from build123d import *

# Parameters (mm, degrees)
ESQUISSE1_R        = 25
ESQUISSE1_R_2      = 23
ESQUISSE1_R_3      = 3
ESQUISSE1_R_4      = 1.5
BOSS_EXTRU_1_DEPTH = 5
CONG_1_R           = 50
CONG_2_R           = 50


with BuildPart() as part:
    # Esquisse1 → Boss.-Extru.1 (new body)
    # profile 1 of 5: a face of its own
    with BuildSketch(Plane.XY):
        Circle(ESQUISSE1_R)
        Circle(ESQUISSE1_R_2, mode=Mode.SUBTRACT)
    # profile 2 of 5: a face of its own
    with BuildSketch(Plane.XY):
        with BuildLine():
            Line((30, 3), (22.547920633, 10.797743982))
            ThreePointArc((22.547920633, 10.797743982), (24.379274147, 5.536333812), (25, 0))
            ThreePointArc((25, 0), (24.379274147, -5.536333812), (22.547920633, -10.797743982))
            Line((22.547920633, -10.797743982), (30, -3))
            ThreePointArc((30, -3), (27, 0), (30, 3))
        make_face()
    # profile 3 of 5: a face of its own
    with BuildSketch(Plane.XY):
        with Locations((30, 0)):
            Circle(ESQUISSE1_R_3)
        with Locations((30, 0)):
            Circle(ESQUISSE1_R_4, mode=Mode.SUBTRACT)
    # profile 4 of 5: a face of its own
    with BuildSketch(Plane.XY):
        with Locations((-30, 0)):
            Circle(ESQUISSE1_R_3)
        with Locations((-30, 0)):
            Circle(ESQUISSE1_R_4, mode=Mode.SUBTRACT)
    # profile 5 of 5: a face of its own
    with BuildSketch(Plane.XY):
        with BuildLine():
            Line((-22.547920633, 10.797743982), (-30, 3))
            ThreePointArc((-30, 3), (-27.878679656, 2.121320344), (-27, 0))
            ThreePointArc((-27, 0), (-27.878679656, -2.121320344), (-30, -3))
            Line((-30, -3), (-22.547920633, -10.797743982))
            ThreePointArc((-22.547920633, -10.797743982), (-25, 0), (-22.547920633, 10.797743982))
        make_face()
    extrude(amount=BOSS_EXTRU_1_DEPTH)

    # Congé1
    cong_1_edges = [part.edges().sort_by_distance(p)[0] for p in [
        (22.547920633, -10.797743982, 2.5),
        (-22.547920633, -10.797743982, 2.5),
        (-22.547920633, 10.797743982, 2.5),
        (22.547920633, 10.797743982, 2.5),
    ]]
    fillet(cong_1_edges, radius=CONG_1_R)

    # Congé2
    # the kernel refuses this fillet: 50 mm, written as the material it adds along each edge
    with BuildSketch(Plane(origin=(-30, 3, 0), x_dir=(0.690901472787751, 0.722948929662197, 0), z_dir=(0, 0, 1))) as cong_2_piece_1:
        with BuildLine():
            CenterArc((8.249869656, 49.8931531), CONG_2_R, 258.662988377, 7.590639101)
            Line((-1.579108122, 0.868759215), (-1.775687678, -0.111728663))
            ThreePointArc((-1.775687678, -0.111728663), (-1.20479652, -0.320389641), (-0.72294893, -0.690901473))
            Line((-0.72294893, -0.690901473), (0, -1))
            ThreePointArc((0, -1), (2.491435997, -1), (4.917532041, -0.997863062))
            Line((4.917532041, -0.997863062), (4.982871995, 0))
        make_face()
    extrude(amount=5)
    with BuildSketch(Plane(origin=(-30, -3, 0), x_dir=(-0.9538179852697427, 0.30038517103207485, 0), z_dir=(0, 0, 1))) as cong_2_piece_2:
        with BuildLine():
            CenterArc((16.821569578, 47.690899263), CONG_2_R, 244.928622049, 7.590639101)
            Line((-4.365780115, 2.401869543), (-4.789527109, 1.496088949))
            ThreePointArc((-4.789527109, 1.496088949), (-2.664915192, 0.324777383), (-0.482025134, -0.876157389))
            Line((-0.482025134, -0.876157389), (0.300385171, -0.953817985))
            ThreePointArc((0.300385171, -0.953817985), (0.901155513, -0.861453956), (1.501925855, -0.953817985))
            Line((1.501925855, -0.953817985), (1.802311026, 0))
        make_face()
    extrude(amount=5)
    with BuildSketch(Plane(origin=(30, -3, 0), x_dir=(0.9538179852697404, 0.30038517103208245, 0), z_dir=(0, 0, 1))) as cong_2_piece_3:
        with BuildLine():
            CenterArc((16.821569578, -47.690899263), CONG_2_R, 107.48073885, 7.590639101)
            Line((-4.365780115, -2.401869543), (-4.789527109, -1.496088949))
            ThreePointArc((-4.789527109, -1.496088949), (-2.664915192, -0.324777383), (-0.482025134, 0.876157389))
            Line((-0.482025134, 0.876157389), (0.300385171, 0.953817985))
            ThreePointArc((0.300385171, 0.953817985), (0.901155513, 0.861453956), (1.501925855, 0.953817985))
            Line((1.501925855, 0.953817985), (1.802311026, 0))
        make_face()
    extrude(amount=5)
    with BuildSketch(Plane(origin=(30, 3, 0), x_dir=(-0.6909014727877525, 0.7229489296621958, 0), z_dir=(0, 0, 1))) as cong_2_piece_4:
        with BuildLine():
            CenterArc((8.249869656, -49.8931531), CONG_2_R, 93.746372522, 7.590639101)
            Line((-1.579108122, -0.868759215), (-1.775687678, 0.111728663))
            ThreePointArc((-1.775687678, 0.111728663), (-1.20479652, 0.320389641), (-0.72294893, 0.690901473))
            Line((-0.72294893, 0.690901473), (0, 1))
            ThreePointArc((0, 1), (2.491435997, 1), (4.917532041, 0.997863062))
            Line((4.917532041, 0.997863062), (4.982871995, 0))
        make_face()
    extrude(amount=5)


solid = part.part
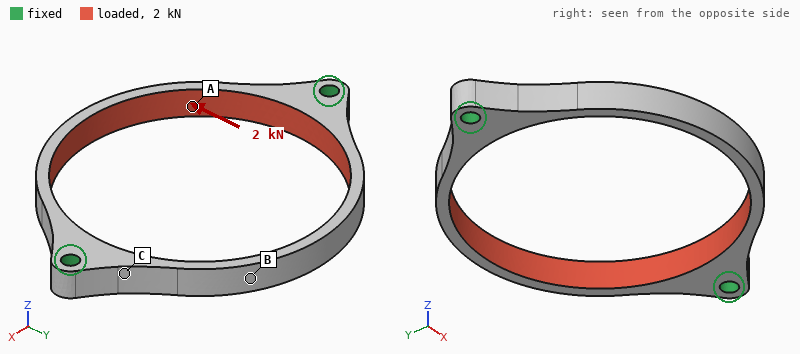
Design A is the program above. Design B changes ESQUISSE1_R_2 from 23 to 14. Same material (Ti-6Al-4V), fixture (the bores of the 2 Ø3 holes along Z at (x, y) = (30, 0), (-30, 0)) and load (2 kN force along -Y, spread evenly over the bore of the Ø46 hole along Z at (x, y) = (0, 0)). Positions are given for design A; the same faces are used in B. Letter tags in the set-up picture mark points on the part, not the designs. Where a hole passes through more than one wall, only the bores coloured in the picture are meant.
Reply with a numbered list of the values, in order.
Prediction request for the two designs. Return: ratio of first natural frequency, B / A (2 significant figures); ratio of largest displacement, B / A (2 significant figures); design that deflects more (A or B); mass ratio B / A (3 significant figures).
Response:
1. 0.82
2. 0.26
3. A
4. 3.27
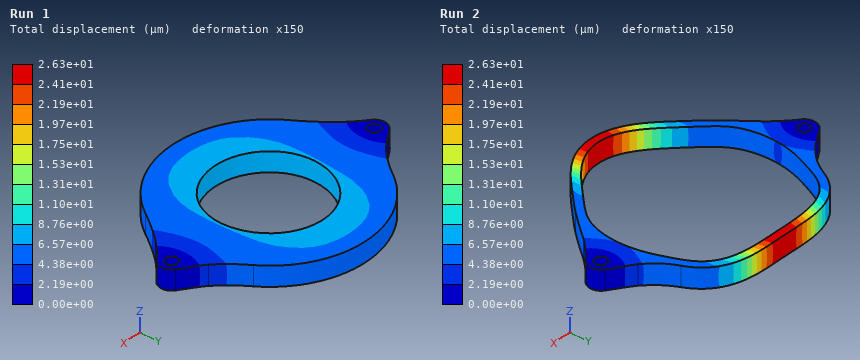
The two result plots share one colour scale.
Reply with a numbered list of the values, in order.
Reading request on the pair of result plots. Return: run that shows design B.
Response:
1. Run 1
